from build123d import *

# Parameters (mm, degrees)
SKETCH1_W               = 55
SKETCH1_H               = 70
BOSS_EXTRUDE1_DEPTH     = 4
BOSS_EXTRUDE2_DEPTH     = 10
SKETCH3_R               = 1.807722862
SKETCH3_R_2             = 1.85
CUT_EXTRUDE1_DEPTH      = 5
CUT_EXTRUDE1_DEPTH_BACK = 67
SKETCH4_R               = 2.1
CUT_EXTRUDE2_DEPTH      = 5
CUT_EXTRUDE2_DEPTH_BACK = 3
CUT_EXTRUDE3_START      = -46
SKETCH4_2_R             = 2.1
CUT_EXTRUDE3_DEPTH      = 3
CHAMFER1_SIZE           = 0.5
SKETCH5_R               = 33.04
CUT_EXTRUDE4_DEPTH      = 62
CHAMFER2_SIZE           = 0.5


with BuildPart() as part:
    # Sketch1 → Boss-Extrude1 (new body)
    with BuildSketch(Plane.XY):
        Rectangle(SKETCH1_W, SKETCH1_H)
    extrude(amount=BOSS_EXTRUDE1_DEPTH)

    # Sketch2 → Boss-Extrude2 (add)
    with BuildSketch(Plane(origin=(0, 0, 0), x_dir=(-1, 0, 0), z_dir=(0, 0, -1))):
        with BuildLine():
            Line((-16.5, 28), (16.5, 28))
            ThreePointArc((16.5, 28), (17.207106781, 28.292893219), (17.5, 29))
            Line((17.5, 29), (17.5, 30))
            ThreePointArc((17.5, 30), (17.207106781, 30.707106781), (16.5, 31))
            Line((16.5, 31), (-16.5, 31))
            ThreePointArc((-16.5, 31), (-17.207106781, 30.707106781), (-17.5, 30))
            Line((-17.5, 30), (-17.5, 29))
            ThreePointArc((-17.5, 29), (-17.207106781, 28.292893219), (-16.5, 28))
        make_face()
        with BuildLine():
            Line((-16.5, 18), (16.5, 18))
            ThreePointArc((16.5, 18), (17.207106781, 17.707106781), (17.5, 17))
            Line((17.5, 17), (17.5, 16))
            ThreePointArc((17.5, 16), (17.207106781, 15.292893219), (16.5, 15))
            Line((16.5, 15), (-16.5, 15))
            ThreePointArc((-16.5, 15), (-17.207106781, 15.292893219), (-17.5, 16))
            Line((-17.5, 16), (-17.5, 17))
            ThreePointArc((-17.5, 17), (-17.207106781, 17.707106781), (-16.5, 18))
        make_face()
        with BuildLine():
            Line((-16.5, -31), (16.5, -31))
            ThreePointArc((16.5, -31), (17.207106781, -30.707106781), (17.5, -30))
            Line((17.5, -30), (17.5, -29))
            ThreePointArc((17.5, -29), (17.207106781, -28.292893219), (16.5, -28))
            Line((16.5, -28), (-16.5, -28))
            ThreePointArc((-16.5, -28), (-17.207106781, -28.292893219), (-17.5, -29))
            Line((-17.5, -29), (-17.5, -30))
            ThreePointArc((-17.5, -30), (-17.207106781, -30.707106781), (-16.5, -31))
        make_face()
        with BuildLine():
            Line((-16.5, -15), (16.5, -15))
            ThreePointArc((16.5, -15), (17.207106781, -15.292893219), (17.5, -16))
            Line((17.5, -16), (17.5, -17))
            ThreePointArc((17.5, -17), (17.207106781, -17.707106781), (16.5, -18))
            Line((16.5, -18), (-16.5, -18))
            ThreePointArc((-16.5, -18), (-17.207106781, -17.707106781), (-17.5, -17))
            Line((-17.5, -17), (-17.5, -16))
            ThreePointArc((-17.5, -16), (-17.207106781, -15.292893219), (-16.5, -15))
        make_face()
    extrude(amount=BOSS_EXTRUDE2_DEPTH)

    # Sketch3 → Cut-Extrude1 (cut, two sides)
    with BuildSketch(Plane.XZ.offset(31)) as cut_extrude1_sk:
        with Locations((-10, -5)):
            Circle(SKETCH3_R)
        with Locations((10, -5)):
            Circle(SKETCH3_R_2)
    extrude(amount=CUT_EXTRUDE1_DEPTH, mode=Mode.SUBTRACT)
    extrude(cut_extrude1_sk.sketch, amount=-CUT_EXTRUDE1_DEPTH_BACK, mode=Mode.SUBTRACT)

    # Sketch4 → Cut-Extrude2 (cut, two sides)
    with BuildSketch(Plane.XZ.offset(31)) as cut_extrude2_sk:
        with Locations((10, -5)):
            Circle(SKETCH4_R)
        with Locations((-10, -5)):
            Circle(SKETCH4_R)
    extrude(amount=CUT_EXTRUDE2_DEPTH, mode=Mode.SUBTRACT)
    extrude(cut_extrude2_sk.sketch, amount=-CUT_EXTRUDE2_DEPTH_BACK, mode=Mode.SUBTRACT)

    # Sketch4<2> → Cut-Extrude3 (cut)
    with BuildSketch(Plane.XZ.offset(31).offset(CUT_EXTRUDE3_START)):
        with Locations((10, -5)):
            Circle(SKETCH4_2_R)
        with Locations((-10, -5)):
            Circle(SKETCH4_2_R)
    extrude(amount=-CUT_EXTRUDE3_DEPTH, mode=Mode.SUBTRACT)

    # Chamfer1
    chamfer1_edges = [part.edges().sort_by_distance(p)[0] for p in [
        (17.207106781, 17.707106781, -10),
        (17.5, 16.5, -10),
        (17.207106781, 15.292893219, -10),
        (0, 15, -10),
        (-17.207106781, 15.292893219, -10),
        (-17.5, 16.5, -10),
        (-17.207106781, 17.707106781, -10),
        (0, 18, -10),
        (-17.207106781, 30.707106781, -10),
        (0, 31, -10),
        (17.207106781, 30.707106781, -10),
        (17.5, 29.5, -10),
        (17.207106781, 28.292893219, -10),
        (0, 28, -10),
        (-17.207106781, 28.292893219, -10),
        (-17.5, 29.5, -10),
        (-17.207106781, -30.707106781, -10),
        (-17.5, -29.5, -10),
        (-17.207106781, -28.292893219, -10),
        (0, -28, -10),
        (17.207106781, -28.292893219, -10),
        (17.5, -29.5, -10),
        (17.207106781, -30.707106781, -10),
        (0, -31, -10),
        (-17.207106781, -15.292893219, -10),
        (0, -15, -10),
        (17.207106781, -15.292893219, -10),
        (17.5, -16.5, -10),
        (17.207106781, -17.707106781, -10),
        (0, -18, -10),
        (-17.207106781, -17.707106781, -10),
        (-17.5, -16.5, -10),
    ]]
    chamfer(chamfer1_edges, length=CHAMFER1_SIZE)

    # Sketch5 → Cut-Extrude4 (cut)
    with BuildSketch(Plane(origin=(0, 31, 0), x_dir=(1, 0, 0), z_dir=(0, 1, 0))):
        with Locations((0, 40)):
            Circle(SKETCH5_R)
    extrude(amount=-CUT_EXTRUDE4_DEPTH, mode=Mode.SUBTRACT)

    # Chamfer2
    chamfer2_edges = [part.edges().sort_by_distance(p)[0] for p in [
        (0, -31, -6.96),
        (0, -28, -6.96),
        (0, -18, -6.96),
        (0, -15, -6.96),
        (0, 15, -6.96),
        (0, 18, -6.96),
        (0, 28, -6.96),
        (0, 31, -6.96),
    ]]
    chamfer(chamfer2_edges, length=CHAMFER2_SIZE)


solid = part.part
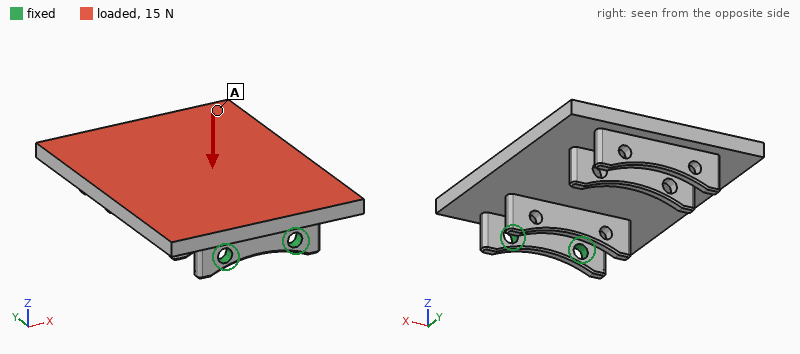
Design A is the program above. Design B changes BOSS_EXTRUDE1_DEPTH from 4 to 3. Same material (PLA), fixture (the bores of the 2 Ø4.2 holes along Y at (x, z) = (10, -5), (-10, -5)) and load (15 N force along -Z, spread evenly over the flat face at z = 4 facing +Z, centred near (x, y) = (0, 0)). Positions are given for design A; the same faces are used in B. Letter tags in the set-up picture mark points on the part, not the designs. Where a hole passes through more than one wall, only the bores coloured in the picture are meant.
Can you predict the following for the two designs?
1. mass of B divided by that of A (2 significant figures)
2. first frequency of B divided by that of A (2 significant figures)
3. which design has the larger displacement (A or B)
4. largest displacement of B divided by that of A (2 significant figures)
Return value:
0.79
0.89
B
1.6
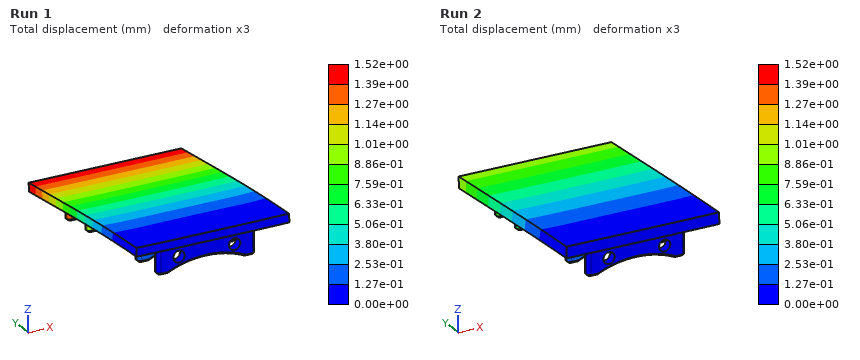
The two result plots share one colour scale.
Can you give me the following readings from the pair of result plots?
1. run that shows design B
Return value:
Run 1
